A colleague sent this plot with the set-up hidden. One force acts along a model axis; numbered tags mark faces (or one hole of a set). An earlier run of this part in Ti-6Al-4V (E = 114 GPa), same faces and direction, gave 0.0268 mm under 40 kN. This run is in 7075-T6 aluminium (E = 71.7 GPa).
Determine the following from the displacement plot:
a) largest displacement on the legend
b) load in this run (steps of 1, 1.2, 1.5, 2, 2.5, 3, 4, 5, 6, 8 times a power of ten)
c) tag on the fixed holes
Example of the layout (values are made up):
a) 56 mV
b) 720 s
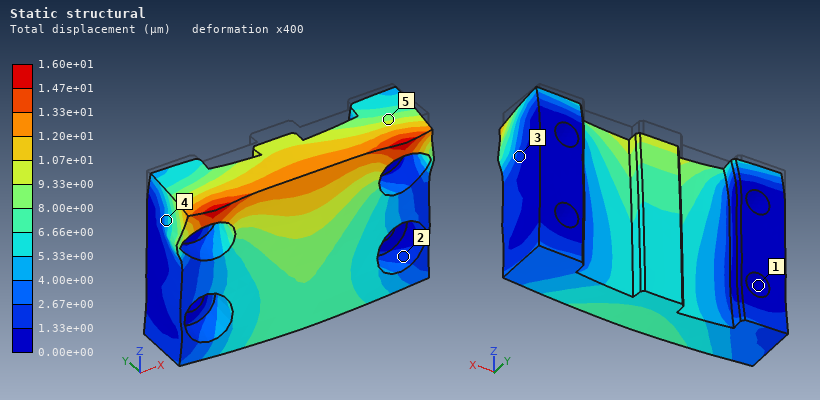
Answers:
a) 1.60e+01 µm
b) 15 kN
c) 1
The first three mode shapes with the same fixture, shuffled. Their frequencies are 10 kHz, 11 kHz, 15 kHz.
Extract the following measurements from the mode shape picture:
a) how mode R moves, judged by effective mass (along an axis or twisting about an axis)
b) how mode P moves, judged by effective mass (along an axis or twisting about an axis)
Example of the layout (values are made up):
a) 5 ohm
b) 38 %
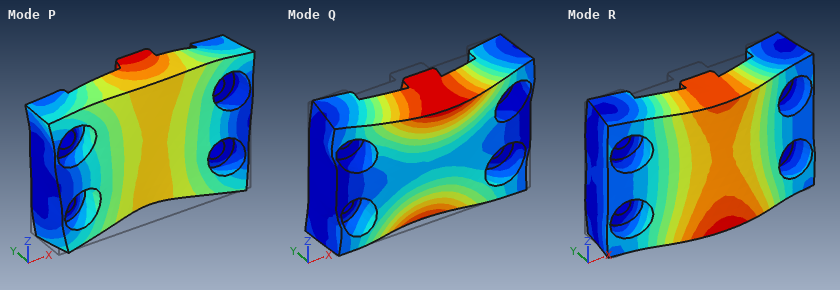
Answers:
a) along Y
b) along Z
